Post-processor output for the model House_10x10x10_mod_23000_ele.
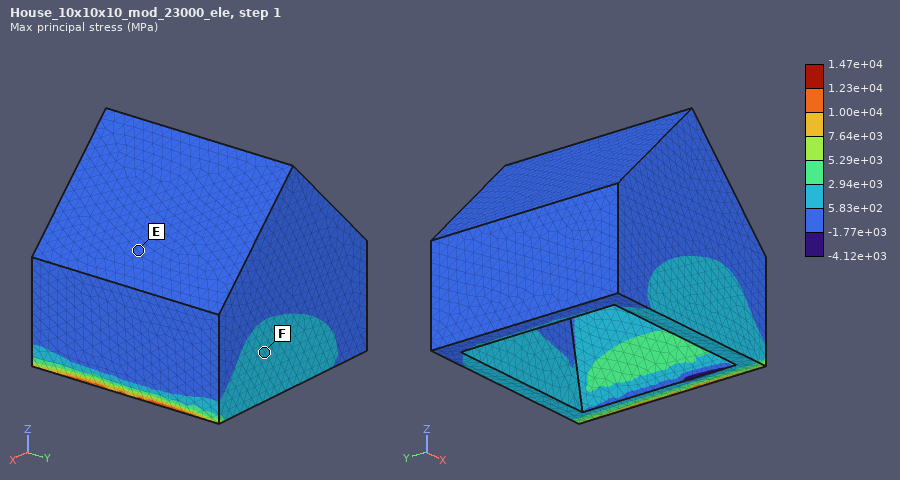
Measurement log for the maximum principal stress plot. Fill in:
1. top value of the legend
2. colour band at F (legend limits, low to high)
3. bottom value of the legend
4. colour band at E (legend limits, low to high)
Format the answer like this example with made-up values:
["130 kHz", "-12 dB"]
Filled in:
["1.47e+04 MPa", "5.83e+02 to 2.94e+03 MPa", "-4.12e+03 MPa", "-1.77e+03 to 5.83e+02 MPa"]
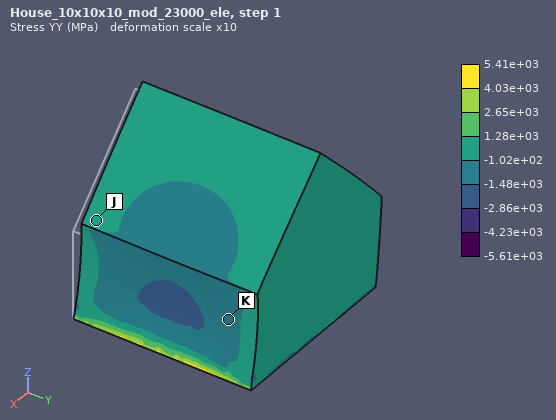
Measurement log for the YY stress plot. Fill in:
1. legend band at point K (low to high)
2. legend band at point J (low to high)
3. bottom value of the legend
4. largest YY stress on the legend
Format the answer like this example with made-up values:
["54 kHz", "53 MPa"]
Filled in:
["-1.48e+03 to -1.02e+02 MPa", "-1.02e+02 to 1.28e+03 MPa", "-5.61e+03 MPa", "5.41e+03 MPa"]
